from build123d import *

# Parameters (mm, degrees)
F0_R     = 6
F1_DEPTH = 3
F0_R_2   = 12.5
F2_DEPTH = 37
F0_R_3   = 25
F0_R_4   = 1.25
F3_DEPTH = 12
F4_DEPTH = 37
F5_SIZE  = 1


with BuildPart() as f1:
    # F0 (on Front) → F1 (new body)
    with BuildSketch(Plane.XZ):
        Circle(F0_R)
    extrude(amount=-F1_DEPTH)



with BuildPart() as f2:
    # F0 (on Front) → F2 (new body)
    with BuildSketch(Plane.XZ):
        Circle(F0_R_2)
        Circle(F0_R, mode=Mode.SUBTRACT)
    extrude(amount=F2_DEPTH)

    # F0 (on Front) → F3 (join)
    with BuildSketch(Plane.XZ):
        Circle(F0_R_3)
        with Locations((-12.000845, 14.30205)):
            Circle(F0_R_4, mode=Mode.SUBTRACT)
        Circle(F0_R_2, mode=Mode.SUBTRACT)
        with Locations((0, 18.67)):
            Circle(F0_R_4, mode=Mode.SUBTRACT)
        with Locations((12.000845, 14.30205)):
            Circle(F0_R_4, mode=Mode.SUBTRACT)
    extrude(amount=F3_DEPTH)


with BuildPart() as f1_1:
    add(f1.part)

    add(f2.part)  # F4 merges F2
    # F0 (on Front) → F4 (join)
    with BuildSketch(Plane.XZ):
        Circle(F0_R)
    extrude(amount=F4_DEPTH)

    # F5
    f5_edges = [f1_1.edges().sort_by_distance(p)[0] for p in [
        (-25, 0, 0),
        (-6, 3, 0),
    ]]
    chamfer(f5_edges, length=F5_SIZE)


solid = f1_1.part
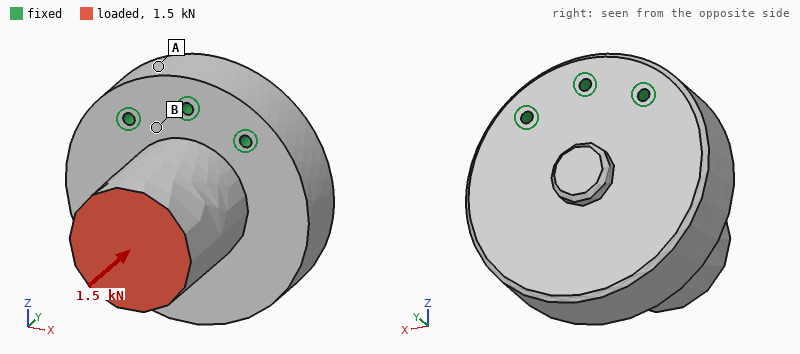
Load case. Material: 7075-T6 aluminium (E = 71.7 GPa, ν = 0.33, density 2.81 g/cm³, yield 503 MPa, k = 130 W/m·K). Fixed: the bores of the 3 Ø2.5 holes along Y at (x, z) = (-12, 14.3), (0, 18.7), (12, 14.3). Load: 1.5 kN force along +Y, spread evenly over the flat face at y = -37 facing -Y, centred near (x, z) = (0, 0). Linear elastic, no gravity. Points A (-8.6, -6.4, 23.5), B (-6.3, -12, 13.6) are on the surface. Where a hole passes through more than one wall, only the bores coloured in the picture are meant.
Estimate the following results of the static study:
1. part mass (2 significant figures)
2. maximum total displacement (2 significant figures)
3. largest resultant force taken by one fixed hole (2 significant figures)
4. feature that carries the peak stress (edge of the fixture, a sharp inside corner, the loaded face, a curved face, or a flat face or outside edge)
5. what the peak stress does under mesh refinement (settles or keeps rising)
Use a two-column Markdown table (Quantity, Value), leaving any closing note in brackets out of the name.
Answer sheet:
| Quantity | Value |
|---|---|
| part mass | 100 g |
| maximum total displacement | 23 µm |
| largest resultant force taken by one fixed hole | 720 N |
| feature that carries the peak stress | edge of the fixture |
| what the peak stress does under mesh refinement | keeps rising |
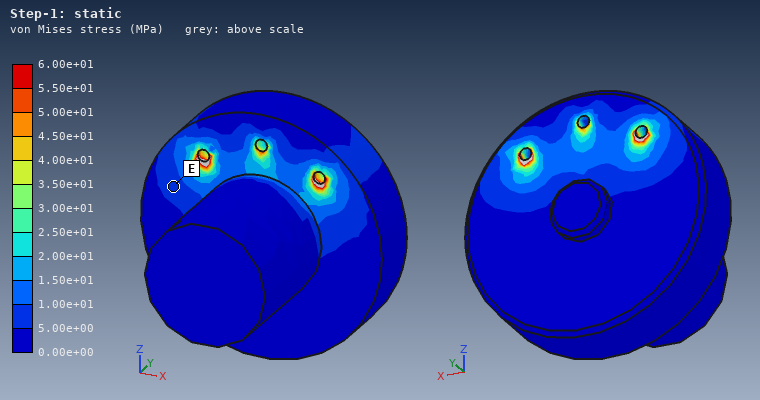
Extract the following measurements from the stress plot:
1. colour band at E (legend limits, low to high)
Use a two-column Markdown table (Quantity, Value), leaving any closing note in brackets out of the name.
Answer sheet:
| Quantity | Value |
|---|---|
| colour band at E | 5.00e+00 to 1.00e+01 MPa |
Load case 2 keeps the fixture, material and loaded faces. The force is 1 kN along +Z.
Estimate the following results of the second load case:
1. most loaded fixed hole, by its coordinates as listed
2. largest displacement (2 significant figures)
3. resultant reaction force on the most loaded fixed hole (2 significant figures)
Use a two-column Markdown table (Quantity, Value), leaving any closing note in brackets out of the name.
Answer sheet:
| Quantity | Value |
|---|---|
| most loaded fixed hole, by its coordinates as listed | (0, 18.7) |
| largest displacement | 43 µm |
| resultant reaction force on the most loaded fixed hole | 770 N |
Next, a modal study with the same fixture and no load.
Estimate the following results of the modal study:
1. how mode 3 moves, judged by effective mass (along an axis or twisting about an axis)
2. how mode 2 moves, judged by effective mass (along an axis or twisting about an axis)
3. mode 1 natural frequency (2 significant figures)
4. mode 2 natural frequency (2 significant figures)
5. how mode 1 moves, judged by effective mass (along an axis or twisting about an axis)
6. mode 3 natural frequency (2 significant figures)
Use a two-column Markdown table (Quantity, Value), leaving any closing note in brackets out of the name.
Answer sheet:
| Quantity | Value |
|---|---|
| how mode 3 moves, judged by effective mass | along X |
| how mode 2 moves, judged by effective mass | along X |
| mode 1 natural frequency | 4500 Hz |
| mode 2 natural frequency | 8700 Hz |
| how mode 1 moves, judged by effective mass | along Y |
| mode 3 natural frequency | 12 kHz |
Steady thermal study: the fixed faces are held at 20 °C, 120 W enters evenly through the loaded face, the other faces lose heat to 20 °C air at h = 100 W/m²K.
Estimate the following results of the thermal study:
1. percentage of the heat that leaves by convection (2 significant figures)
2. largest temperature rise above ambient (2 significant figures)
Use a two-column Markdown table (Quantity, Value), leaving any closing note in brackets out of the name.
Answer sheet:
| Quantity | Value |
|---|---|
| percentage of the heat that leaves by convection | 14 % |
| largest temperature rise above ambient | 70 K |
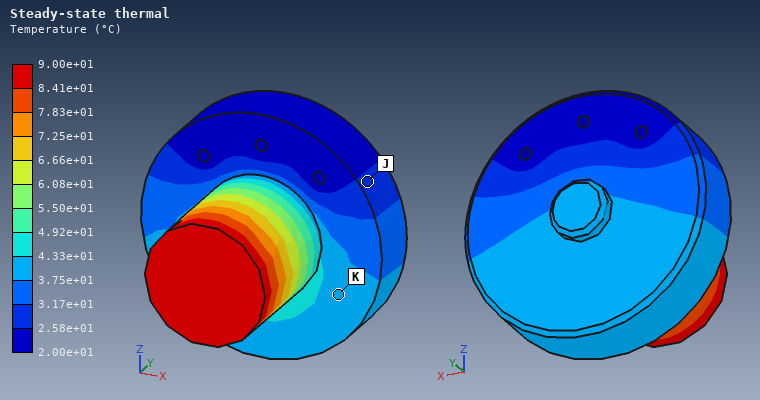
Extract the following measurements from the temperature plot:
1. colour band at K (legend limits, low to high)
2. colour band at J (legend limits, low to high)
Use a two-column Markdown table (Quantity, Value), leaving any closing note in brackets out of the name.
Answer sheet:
| Quantity | Value |
|---|---|
| colour band at K | 3.75e+01 to 4.33e+01 °C |
| colour band at J | 2.58e+01 to 3.17e+01 °C |
